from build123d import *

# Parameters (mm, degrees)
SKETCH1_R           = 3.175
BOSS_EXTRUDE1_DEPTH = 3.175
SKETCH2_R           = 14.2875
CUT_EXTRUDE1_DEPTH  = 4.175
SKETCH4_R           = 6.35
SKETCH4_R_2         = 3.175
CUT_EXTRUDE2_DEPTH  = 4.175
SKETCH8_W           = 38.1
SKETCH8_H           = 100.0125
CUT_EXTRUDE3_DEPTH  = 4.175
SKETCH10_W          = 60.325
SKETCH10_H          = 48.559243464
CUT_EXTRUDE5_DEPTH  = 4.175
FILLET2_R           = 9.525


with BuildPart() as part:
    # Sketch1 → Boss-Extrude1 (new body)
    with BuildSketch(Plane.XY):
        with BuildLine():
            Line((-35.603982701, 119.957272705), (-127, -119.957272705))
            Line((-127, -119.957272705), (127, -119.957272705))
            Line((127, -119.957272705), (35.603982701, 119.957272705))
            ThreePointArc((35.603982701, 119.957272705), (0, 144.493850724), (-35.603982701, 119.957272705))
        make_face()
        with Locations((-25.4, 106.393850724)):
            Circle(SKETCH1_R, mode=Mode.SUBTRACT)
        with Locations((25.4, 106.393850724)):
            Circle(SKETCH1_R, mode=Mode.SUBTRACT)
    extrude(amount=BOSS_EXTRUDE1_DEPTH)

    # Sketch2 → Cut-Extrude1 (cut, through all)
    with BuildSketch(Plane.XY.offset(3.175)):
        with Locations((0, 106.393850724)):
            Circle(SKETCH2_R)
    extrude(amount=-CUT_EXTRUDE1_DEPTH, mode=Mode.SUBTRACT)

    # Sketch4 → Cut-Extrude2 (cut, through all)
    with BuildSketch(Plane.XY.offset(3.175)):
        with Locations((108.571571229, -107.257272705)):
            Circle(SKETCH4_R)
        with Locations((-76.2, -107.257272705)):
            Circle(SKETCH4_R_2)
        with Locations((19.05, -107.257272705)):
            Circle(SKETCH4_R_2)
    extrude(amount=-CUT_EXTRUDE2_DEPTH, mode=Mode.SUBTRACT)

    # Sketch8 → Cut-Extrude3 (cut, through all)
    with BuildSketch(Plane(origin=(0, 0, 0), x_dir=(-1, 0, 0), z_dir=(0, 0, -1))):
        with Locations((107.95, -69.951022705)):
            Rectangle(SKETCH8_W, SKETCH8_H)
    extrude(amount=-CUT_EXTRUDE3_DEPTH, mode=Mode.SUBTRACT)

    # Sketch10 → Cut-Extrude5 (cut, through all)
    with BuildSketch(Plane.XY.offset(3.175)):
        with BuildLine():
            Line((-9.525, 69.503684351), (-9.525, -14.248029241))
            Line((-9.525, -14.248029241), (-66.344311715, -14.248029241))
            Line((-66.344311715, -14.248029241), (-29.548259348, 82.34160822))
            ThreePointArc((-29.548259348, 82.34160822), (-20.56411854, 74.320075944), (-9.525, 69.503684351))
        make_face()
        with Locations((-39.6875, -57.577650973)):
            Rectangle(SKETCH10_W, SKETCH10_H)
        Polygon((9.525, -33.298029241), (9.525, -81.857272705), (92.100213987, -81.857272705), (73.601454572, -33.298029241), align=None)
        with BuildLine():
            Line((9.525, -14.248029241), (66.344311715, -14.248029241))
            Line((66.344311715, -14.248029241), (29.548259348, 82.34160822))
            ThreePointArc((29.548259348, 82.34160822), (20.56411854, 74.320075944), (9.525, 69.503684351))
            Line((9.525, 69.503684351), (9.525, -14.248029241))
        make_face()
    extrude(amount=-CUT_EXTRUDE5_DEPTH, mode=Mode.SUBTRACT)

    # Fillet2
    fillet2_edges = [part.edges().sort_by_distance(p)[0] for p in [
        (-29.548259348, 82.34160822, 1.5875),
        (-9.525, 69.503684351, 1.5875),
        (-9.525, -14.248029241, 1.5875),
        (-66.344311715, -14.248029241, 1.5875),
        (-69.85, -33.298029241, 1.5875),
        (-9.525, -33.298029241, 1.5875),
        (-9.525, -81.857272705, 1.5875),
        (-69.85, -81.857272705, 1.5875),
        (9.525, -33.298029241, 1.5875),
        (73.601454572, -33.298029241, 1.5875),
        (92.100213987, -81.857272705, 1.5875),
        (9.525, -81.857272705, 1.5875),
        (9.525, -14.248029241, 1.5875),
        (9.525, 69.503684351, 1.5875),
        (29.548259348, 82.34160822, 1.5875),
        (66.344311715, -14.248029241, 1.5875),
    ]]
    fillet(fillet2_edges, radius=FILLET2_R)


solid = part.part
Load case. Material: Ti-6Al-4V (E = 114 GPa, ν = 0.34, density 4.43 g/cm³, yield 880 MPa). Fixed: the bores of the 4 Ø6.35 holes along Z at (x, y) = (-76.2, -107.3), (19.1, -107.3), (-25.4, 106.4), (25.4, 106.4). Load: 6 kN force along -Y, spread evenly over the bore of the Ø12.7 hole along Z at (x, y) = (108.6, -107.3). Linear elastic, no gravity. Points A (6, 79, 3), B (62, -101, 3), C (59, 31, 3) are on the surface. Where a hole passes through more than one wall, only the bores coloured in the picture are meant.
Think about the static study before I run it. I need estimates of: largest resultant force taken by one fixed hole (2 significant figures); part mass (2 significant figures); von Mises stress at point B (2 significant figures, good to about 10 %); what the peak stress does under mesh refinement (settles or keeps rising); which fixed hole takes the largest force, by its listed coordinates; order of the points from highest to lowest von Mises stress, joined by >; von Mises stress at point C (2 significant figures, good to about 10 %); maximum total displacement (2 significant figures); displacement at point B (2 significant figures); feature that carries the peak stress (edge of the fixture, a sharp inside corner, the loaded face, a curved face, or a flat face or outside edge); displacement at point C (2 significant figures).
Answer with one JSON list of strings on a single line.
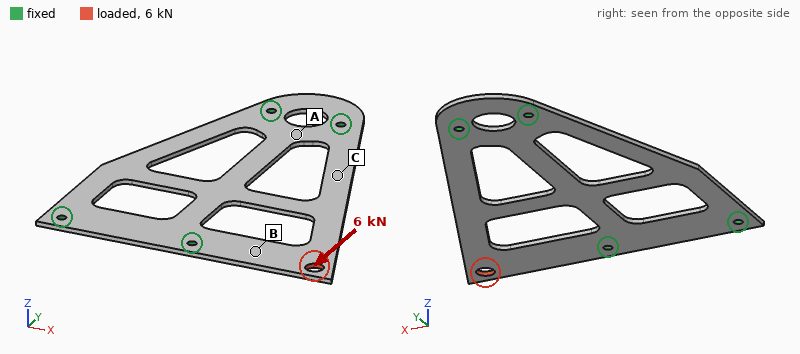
["4.7 kN", "340 g", "29 MPa", "keeps rising", "(25.4, 106.4)", "C > B > A", "79 MPa", "0.22 mm", "0.069 mm", "edge of the fixture", "0.056 mm"]
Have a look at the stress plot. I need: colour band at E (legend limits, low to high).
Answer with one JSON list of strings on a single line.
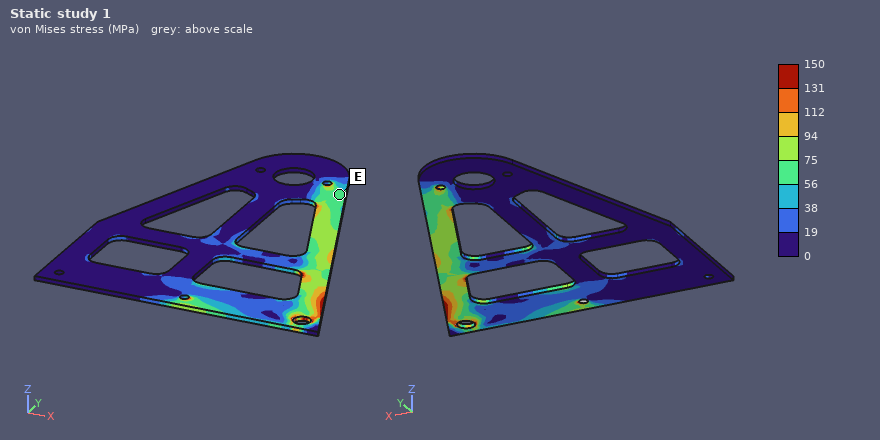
["56 to 75 MPa"]
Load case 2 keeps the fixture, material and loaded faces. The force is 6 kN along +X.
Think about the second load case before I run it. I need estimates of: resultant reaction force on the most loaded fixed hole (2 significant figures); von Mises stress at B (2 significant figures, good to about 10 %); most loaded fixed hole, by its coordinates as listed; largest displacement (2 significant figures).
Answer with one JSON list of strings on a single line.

["5.4 kN", "51 MPa", "(19.1, -107.3)", "76 µm"]
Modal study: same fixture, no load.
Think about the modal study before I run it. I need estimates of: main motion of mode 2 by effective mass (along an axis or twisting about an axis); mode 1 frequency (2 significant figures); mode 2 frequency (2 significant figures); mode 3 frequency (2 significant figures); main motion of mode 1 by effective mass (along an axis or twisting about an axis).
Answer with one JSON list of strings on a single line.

["along Z", "230 Hz", "340 Hz", "410 Hz", "along Z"]
